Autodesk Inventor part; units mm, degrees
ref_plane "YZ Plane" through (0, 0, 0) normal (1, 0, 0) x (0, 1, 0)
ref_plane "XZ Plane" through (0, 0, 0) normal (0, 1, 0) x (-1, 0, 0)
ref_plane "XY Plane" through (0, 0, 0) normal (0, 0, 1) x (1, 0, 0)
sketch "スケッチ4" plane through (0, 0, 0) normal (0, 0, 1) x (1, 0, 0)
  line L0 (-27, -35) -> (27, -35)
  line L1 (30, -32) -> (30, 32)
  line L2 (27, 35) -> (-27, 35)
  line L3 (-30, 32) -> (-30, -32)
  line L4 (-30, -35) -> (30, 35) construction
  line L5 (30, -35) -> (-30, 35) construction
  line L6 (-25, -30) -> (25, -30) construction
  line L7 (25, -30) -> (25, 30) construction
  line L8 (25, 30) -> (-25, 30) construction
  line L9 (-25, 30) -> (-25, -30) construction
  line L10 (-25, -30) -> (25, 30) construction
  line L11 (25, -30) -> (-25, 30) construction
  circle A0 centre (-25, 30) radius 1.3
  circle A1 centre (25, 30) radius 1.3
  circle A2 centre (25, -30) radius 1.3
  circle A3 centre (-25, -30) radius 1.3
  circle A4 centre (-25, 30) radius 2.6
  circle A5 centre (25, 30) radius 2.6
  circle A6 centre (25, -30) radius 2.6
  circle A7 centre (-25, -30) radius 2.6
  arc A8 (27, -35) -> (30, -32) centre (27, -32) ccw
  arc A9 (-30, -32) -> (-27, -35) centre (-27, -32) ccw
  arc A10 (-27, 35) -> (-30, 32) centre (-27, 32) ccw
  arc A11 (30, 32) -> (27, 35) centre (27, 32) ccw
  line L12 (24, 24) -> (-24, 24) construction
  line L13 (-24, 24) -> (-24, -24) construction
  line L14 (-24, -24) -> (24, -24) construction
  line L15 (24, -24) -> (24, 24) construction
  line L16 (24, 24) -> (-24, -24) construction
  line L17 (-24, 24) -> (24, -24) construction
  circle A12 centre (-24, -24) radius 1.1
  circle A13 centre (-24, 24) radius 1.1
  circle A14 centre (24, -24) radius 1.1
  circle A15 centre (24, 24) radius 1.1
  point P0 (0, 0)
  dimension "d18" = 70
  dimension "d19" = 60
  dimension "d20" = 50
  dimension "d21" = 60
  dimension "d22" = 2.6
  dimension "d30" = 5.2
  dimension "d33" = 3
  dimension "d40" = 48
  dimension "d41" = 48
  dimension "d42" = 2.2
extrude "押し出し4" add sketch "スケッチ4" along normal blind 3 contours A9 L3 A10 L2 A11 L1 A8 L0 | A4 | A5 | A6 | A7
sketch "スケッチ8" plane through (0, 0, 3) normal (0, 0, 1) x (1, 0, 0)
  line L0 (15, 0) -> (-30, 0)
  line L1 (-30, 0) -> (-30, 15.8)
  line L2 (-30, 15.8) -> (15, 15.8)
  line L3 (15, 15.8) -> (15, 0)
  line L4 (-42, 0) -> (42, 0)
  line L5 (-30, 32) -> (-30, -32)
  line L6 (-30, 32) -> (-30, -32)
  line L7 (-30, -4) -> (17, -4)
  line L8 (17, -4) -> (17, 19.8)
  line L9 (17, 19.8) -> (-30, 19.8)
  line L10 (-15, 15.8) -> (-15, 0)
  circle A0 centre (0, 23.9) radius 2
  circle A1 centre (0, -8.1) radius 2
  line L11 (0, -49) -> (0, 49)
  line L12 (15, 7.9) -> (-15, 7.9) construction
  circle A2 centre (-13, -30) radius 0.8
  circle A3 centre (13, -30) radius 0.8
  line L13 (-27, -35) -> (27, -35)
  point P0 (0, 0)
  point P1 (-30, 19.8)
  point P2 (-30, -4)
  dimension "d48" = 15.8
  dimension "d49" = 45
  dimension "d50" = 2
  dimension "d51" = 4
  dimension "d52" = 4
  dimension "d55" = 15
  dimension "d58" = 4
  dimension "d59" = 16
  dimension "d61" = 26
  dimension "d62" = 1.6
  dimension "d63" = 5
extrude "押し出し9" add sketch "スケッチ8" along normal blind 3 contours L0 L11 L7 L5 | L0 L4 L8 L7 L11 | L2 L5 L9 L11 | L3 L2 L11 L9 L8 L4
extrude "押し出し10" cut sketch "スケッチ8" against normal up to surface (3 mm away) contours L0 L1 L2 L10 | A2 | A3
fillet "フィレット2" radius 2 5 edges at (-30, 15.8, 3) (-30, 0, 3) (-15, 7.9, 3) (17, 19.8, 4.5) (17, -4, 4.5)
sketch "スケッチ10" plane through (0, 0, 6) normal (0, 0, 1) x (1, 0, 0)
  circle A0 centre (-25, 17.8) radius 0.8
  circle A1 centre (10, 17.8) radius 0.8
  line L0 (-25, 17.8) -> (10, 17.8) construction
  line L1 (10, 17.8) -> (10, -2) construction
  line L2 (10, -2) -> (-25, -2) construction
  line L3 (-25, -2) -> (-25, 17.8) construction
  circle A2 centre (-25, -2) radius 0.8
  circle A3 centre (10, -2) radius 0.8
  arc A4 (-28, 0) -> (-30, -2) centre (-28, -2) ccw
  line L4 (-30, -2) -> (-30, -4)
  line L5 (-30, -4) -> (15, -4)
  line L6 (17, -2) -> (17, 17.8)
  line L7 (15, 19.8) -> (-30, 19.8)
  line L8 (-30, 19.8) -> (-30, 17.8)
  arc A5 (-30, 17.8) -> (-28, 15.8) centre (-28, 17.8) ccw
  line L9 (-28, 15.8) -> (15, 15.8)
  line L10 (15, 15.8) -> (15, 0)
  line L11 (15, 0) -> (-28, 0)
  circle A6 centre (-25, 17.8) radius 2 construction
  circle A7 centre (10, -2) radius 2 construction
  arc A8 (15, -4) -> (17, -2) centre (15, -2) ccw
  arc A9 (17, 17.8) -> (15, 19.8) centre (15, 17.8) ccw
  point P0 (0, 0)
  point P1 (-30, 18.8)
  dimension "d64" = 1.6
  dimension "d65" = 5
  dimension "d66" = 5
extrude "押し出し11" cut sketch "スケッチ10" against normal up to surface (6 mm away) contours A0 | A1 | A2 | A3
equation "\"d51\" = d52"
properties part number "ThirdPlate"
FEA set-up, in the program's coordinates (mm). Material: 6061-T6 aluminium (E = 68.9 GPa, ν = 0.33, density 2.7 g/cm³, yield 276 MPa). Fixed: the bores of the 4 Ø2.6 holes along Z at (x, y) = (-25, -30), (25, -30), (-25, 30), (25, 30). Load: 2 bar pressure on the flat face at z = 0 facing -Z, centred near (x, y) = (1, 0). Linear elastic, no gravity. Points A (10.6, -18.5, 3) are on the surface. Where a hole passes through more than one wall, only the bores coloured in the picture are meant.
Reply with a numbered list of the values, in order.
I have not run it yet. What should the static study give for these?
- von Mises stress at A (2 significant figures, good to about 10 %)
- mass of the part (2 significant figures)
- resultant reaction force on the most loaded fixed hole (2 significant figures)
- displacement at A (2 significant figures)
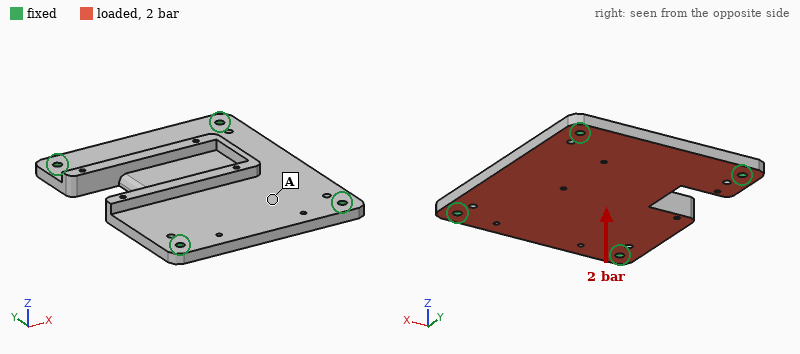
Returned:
1. 13 MPa
2. 35 g
3. 210 N
4. 51 µm
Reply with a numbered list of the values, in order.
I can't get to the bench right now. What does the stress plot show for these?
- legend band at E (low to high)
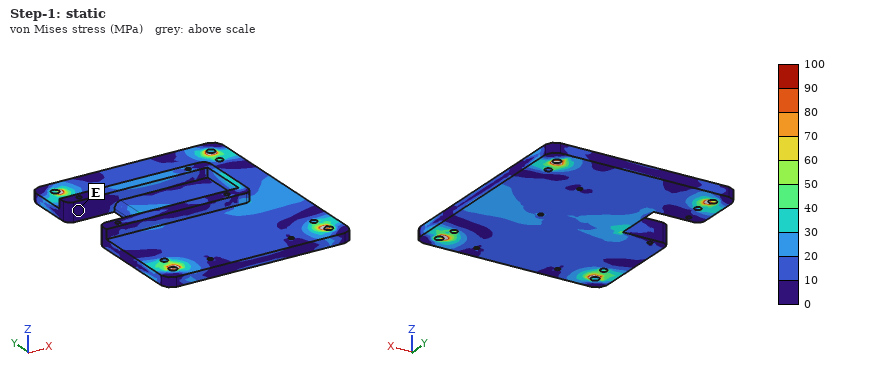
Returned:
1. 0 to 10 MPa
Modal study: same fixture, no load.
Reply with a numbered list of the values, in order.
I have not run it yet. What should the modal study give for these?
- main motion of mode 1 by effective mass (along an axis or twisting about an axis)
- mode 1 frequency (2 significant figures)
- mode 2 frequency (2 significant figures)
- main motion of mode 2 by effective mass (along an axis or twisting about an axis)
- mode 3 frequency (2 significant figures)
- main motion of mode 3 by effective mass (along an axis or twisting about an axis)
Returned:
1. along Z
2. 3000 Hz
3. 4800 Hz
4. twisting about Y
5. 6200 Hz
6. twisting about X
